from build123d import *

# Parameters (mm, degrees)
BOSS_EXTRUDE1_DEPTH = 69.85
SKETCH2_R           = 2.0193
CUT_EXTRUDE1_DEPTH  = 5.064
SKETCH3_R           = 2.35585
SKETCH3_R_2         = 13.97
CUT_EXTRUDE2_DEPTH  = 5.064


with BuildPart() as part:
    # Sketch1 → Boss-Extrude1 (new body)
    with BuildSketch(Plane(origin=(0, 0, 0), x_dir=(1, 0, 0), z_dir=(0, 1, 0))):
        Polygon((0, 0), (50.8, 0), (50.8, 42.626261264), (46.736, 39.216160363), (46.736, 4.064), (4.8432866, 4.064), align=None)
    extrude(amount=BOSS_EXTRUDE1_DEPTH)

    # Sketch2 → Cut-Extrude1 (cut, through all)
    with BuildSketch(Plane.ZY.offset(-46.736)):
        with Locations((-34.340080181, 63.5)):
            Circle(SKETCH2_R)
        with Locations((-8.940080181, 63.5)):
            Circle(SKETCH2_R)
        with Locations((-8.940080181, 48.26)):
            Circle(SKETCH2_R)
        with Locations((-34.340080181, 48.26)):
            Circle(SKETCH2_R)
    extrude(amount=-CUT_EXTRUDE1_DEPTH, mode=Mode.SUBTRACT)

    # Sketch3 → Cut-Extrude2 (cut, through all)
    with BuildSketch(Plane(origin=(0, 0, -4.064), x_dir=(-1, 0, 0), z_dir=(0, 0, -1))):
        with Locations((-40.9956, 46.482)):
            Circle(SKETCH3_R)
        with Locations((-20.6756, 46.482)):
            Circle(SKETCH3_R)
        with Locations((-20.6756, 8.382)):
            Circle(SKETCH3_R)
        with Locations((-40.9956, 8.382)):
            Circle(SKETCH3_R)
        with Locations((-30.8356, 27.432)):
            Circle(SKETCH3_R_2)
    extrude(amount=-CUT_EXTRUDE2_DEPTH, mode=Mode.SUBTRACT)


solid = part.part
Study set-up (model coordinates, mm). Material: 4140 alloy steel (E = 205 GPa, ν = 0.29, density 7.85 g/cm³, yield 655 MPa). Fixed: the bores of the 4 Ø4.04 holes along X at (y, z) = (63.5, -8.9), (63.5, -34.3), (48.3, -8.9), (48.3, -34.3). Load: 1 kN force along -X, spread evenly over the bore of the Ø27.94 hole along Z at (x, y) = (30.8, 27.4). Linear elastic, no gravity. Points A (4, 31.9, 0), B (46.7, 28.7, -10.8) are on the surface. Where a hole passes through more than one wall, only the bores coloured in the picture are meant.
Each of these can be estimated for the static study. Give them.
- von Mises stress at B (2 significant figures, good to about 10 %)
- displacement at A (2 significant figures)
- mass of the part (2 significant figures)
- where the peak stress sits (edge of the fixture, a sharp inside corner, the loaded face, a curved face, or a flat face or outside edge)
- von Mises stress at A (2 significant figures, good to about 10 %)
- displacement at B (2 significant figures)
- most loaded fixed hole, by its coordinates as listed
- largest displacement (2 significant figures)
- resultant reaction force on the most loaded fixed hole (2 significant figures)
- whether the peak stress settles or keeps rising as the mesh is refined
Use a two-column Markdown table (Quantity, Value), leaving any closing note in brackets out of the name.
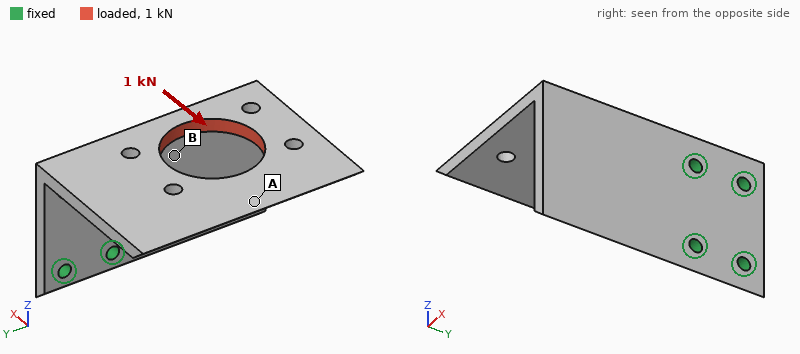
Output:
| Quantity | Value |
|---|---|
| von Mises stress at B | 20 MPa |
| displacement at A | 62 µm |
| mass of the part | 170 g |
| where the peak stress sits | edge of the fixture |
| von Mises stress at A | 11 MPa |
| displacement at B | 20 µm |
| most loaded fixed hole, by its coordinates as listed | (48.3, -8.9) |
| largest displacement | 91 µm |
| resultant reaction force on the most loaded fixed hole | 2.0 kN |
| whether the peak stress settles or keeps rising as the mesh is refined | keeps rising |
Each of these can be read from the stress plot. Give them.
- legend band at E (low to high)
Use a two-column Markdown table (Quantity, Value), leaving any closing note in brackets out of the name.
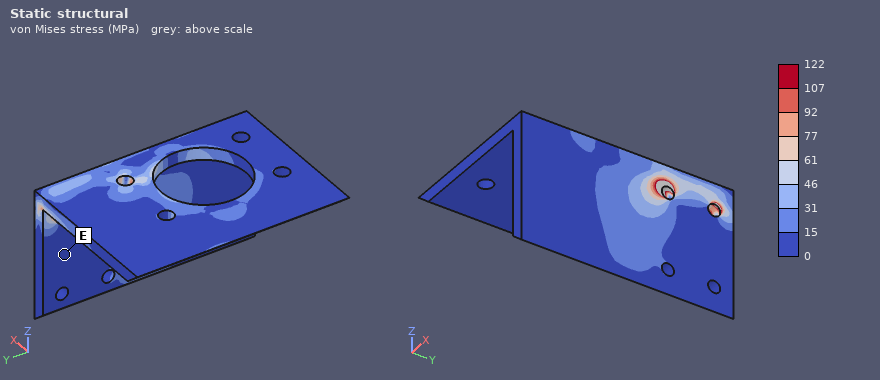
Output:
| Quantity | Value |
|---|---|
| legend band at E | 0 to 15 MPa |
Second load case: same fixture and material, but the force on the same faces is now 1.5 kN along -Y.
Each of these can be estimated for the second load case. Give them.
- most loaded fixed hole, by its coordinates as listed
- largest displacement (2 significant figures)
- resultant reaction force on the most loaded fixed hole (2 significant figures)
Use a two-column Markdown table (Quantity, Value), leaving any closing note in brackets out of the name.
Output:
| Quantity | Value |
|---|---|
| most loaded fixed hole, by its coordinates as listed | (48.3, -8.9) |
| largest displacement | 68 µm |
| resultant reaction force on the most loaded fixed hole | 1.7 kN |
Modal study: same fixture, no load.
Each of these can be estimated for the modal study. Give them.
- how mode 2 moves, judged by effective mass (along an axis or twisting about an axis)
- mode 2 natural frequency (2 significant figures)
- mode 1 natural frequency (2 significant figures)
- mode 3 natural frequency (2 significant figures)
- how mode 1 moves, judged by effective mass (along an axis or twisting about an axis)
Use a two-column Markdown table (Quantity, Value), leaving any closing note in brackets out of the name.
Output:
| Quantity | Value |
|---|---|
| how mode 2 moves, judged by effective mass | along X |
| mode 2 natural frequency | 2000 Hz |
| mode 1 natural frequency | 1000 Hz |
| mode 3 natural frequency | 2100 Hz |
| how mode 1 moves, judged by effective mass | along Z |
